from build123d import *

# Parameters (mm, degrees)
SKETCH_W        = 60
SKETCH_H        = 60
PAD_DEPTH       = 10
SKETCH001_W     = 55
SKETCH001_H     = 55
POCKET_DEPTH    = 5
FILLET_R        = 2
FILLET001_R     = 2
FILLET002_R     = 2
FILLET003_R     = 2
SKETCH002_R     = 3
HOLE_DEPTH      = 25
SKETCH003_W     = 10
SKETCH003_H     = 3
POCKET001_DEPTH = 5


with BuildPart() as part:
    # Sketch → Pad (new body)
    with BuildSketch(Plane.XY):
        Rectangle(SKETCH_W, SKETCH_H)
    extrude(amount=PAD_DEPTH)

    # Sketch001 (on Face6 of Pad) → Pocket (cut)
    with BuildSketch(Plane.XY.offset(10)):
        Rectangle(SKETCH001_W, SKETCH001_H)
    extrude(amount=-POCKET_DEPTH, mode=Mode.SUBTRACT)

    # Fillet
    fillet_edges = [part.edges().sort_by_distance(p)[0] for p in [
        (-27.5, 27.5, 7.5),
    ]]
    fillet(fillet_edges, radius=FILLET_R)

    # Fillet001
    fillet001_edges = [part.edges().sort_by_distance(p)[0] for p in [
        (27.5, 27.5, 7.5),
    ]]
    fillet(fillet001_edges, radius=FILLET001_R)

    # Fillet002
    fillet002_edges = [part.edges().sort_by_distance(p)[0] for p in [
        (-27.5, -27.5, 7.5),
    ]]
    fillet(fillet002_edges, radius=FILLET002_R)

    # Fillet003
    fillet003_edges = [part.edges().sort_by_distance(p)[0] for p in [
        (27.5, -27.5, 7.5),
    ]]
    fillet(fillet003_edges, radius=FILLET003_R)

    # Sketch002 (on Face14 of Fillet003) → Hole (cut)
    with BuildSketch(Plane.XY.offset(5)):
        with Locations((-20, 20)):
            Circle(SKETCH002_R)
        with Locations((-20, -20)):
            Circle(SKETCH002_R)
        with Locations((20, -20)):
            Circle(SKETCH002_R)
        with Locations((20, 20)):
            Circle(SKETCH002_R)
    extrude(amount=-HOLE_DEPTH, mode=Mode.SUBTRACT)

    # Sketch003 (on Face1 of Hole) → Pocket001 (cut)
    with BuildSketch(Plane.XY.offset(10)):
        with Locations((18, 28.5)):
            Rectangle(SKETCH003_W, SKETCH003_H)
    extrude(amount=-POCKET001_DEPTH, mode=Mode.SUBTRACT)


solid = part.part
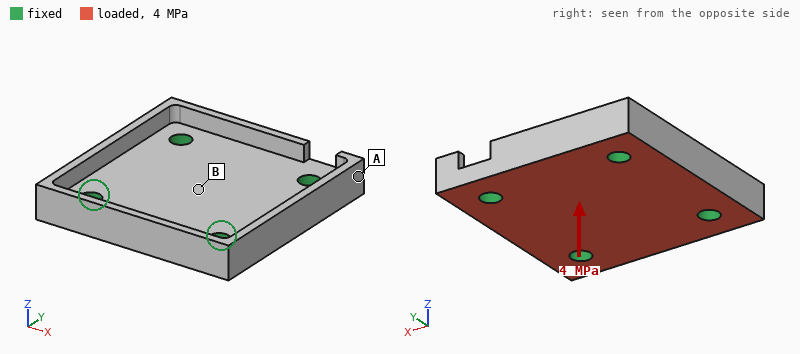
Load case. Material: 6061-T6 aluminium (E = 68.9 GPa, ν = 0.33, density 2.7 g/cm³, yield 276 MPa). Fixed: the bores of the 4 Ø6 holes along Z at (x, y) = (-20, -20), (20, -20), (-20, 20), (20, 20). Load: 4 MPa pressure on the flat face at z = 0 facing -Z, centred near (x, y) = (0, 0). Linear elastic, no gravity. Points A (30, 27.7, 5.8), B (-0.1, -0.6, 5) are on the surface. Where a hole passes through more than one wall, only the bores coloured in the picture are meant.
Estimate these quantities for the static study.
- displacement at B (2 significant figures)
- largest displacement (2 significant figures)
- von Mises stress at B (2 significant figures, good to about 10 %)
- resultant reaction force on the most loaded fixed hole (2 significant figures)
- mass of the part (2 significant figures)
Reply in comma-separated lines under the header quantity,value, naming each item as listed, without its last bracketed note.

quantity,value
displacement at B,71 µm
largest displacement,71 µm
von Mises stress at B,64 MPa
resultant reaction force on the most loaded fixed hole,3.5 kN
mass of the part,55 g
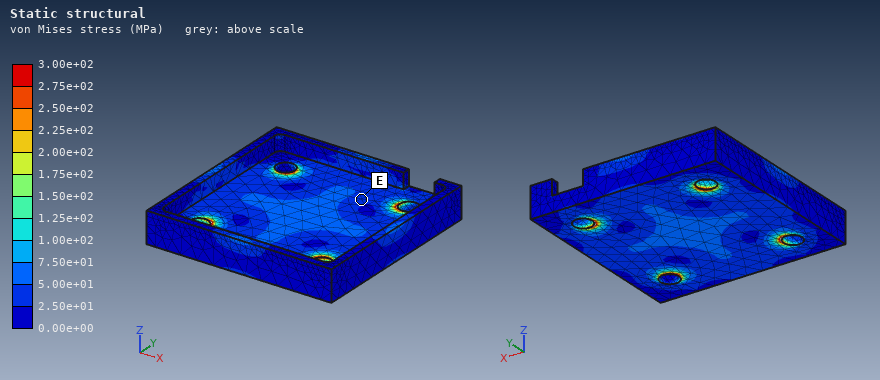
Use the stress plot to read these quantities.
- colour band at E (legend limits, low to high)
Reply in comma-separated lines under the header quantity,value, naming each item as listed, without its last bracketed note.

quantity,value
colour band at E,2.50e+01 to 5.00e+01 MPa
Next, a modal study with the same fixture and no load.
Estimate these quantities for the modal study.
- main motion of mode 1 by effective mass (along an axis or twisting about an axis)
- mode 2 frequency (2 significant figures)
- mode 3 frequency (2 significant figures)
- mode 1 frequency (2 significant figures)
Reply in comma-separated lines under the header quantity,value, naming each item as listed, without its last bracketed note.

quantity,value
main motion of mode 1 by effective mass,along Z
mode 2 frequency,17 kHz
mode 3 frequency,17 kHz
mode 1 frequency,12 kHz
